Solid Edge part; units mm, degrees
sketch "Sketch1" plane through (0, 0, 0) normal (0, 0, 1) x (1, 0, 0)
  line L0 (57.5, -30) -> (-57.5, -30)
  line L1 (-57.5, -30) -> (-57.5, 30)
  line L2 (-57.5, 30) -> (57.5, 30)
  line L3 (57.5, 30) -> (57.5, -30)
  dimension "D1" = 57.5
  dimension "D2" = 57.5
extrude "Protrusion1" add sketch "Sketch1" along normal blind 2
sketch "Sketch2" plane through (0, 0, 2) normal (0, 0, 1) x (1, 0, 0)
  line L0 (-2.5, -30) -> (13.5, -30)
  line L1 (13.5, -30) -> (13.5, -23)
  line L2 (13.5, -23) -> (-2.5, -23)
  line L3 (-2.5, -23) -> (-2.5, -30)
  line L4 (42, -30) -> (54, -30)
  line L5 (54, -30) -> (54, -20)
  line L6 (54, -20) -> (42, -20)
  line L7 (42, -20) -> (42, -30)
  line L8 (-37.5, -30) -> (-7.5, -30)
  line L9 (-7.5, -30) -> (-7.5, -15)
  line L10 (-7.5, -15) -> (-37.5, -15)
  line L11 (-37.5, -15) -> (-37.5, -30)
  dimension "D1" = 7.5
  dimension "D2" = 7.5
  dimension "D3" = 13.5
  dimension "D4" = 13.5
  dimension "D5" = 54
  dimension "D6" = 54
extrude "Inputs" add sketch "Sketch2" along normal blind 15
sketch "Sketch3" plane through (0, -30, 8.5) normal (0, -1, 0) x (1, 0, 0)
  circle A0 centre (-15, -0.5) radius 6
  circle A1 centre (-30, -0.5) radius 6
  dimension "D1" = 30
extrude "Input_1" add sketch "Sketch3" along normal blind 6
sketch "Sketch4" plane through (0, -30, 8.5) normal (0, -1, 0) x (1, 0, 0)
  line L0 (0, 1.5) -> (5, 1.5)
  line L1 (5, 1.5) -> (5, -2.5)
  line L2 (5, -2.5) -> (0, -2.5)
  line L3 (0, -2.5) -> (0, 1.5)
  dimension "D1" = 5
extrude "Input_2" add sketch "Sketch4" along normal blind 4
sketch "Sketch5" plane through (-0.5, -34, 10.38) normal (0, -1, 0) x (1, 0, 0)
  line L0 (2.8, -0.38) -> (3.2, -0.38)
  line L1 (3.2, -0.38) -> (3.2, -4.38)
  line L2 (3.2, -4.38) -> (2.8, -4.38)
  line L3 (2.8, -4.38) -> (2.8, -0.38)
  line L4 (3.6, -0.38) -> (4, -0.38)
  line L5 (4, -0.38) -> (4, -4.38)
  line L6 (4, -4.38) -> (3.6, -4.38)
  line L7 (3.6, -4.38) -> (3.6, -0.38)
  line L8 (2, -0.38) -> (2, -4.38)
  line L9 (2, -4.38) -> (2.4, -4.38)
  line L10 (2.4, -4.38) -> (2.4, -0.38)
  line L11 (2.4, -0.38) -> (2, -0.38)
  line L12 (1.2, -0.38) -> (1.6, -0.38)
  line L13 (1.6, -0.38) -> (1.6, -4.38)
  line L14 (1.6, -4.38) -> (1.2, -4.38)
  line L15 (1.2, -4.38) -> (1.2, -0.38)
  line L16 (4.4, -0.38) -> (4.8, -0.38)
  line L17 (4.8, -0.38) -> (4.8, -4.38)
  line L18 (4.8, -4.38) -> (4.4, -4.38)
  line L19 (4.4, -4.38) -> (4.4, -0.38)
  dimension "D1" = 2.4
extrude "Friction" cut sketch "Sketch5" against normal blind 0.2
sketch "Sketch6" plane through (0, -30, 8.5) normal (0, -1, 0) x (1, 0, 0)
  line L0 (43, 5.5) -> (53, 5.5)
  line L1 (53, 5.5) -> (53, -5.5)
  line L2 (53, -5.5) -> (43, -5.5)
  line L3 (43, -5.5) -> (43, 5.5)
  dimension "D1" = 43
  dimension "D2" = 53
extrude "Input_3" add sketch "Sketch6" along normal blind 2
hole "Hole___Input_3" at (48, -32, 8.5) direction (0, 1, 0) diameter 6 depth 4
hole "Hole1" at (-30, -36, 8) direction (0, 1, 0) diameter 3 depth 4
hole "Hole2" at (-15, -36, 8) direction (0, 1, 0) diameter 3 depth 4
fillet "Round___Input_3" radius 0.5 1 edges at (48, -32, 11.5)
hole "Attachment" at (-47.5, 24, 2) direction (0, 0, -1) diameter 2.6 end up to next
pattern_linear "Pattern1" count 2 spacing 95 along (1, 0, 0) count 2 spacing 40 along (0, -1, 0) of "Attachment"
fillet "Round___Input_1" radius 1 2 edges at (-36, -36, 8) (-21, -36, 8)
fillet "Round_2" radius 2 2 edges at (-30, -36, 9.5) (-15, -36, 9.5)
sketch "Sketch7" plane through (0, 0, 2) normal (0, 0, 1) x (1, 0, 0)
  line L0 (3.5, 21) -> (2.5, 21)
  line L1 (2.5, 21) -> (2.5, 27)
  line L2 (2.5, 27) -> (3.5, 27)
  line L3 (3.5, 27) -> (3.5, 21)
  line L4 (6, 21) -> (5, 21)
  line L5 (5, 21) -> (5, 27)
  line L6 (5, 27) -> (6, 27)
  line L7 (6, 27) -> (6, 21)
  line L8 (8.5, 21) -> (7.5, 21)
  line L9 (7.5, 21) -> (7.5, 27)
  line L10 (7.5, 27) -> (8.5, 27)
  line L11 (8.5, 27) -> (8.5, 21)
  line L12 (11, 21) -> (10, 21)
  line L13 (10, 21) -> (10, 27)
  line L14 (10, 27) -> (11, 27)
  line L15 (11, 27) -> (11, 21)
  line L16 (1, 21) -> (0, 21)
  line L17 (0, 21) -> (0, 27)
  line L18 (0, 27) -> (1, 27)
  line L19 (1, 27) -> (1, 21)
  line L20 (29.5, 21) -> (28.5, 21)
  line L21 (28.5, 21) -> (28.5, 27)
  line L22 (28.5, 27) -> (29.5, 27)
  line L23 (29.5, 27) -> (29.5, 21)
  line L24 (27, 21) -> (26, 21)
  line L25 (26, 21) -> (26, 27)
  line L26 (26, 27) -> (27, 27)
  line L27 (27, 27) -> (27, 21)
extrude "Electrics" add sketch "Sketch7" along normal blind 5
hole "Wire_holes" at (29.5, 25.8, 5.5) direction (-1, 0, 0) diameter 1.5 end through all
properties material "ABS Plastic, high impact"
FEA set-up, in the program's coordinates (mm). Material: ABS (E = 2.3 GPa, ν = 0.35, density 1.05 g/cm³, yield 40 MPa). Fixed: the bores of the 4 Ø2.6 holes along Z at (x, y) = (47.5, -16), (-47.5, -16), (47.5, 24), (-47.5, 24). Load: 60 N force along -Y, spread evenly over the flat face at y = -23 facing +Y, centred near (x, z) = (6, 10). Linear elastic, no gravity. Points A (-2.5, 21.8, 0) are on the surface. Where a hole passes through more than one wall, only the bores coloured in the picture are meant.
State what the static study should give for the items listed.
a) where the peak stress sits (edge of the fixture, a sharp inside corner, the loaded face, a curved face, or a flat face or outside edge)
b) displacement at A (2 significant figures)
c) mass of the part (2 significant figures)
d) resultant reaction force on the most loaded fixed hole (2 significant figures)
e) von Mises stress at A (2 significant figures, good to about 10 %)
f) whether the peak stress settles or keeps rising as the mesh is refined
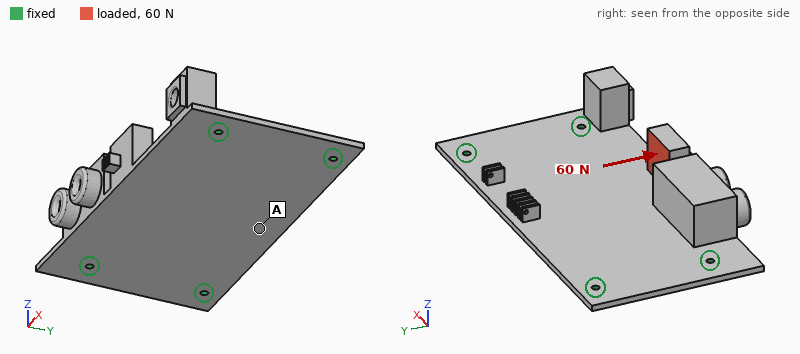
edge of the fixture
0.36 mm
27 g
23 N
1.5 MPa
keeps rising
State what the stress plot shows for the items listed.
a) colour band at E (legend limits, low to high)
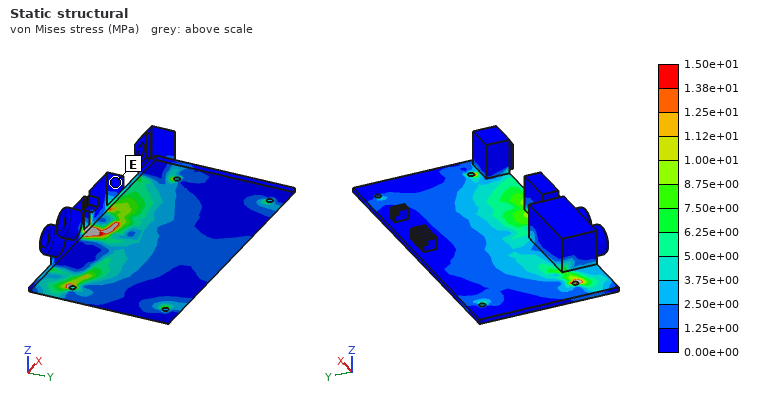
0.00e+00 to 1.25e+00 MPa
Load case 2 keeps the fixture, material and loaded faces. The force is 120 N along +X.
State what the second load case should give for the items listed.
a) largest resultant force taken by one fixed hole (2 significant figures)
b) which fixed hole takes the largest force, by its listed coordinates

58 N
(-47.5, -16)
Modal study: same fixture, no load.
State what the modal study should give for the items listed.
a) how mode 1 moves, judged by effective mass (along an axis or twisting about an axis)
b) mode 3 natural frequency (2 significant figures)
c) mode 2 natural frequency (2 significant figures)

along Z
630 Hz
350 Hz
